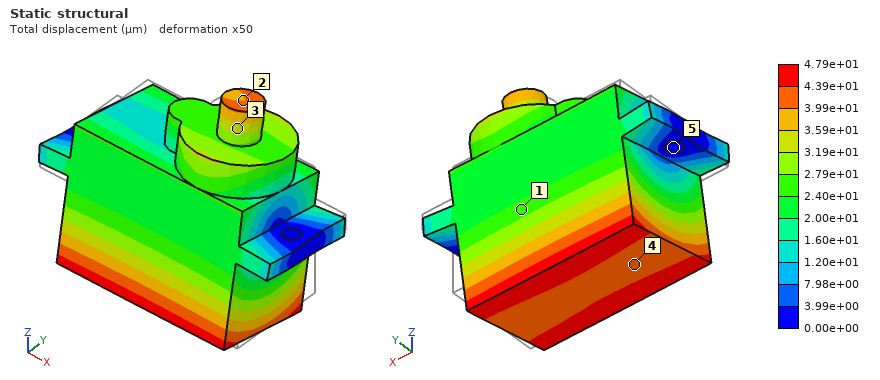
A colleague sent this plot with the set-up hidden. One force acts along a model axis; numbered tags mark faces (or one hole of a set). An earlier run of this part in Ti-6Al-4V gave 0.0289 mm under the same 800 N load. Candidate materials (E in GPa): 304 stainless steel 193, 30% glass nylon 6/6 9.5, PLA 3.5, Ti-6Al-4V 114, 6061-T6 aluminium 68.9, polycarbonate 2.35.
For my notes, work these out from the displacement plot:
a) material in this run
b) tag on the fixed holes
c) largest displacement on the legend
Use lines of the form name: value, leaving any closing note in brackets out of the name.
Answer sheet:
material in this run: 6061-T6 aluminium
tag on the fixed holes: 5
largest displacement on the legend: 4.79e+01 µm
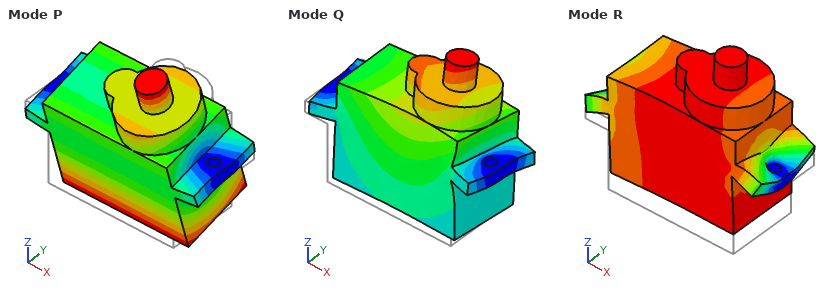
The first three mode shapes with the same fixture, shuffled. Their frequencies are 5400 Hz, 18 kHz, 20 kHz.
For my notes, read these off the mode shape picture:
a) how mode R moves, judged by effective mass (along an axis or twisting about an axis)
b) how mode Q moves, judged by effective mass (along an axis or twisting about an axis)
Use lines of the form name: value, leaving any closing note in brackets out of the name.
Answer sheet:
how mode R moves, judged by effective mass: along Z
how mode Q moves, judged by effective mass: along Y
